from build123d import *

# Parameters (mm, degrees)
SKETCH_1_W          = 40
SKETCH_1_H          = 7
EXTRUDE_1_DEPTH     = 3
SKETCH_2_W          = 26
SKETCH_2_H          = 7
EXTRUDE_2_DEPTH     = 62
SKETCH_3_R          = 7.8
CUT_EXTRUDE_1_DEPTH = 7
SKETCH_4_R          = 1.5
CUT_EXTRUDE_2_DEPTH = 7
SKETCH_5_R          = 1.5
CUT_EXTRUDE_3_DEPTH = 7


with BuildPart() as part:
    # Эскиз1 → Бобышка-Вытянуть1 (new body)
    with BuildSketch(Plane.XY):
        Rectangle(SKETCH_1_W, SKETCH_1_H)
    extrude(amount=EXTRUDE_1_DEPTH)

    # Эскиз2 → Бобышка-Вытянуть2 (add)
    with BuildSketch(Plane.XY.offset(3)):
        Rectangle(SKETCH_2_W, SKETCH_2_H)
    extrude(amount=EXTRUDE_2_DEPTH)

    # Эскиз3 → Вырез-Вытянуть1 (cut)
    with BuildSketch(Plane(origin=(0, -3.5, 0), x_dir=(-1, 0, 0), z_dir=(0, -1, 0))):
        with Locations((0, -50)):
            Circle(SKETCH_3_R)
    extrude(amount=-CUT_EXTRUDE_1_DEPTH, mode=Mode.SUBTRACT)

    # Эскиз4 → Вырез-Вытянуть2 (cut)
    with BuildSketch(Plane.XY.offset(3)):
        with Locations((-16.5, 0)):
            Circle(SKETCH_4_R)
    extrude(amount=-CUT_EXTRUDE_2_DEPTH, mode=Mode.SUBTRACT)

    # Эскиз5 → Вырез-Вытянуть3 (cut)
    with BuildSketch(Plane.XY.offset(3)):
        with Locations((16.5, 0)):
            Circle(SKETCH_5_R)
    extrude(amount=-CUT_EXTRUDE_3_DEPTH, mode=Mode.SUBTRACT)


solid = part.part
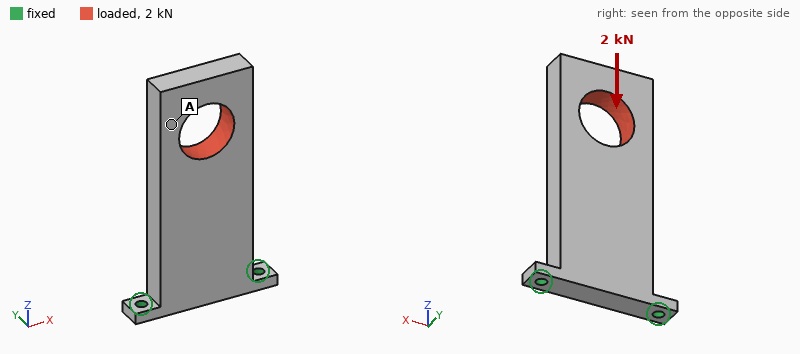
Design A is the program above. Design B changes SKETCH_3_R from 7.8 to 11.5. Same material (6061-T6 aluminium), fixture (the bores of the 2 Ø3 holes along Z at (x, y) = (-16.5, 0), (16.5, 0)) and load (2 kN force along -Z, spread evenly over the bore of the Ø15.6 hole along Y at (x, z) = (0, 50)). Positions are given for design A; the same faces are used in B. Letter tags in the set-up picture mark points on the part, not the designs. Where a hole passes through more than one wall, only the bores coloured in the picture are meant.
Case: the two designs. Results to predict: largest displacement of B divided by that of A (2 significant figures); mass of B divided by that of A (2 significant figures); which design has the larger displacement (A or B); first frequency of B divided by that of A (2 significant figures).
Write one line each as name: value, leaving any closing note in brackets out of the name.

largest displacement of B divided by that of A: 2.4
mass of B divided by that of A: 0.85
which design has the larger displacement: B
first frequency of B divided by that of A: 1.2
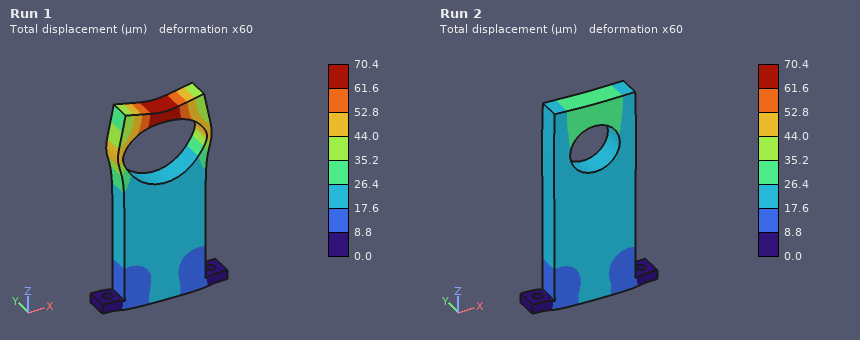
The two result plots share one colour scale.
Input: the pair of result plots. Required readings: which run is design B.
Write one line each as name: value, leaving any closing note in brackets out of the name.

which run is design B: Run 1
